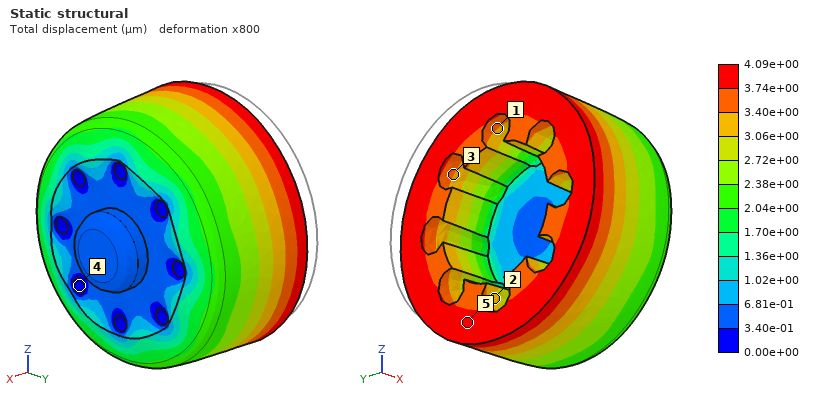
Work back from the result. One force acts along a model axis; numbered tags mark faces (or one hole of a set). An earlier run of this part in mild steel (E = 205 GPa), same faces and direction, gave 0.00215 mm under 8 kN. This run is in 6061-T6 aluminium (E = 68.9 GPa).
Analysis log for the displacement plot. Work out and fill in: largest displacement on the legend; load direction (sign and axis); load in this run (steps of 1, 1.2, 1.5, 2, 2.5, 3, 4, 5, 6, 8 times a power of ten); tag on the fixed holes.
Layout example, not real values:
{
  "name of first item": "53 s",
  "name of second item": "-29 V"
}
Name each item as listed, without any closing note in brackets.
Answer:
{
  "largest displacement on the legend": "4.09e+00 µm",
  "load direction": "+X",
  "load in this run": "5 kN",
  "tag on the fixed holes": "4"
}
